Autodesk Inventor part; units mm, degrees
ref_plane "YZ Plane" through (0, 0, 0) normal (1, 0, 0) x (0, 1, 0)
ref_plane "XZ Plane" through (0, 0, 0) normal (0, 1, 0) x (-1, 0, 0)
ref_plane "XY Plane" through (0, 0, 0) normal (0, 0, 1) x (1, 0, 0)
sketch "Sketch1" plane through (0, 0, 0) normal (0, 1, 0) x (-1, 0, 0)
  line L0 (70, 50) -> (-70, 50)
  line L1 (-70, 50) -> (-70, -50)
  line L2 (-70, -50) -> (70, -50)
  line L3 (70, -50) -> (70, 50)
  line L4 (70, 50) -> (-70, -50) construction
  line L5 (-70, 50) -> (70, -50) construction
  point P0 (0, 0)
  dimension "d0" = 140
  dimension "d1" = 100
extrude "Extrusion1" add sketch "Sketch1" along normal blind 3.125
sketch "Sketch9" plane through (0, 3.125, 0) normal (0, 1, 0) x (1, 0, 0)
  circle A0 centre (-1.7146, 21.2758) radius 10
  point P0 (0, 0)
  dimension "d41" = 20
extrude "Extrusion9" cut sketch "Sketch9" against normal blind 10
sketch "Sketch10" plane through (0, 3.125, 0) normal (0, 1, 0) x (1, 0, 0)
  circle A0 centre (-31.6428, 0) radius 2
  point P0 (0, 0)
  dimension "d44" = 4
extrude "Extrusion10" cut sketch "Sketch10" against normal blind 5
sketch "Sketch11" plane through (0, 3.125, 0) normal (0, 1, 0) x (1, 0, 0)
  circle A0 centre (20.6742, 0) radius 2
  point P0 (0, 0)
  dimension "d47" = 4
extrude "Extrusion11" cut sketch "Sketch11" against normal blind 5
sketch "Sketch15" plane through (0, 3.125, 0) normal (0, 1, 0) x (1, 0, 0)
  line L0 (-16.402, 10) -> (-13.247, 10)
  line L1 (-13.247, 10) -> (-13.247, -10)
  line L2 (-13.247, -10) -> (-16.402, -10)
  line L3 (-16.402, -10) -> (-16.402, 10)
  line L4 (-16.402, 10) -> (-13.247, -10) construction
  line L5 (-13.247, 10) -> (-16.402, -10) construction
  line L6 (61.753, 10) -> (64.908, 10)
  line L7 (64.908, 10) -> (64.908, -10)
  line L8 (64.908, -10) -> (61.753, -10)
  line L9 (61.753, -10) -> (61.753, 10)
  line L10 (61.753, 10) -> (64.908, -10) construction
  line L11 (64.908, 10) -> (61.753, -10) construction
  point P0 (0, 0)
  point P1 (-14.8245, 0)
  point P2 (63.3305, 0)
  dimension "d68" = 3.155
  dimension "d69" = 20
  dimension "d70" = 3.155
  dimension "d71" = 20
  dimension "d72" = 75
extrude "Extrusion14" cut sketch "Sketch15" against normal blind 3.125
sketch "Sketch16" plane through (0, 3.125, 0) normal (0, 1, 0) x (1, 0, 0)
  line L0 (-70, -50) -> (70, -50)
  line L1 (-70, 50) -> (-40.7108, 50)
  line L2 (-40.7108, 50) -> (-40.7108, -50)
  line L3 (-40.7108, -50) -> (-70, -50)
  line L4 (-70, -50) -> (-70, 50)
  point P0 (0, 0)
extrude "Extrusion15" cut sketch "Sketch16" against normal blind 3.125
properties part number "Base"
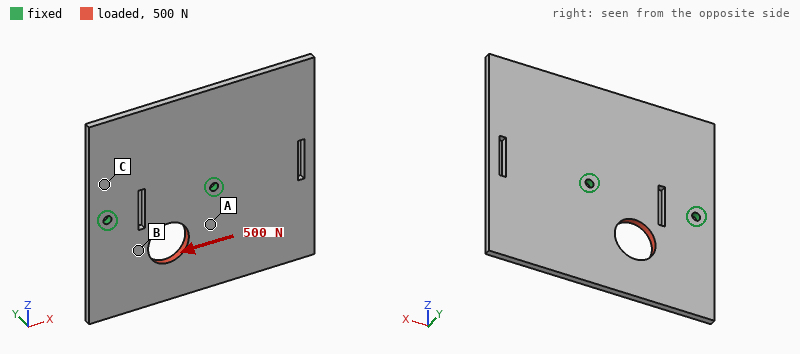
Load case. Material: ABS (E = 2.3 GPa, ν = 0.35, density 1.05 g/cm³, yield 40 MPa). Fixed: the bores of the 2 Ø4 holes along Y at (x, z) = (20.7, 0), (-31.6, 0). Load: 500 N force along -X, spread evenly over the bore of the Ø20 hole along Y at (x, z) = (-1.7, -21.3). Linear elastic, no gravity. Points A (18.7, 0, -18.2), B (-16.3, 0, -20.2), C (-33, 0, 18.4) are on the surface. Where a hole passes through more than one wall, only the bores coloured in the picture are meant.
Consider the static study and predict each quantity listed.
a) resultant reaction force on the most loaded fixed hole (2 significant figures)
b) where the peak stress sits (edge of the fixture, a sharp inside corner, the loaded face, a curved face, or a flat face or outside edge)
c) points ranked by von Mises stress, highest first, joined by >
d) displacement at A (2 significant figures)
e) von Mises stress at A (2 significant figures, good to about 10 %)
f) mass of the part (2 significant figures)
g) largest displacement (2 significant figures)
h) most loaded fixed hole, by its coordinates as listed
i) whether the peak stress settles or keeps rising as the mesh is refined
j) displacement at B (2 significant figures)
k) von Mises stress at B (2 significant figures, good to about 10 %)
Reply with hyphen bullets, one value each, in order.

- 390 N
- edge of the fixture
- B > A > C
- 0.079 mm
- 3.0 MPa
- 35 g
- 0.18 mm
- (20.7, 0)
- keeps rising
- 0.088 mm
- 4.8 MPa
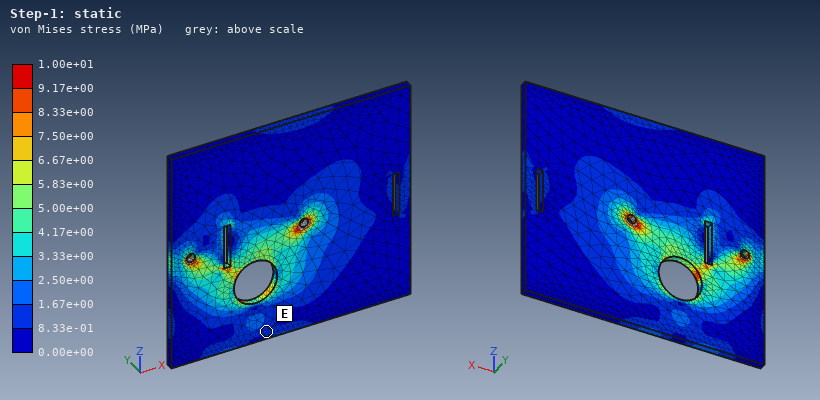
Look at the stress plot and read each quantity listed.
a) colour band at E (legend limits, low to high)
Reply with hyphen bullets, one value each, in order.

- 8.33e-01 to 1.67e+00 MPa
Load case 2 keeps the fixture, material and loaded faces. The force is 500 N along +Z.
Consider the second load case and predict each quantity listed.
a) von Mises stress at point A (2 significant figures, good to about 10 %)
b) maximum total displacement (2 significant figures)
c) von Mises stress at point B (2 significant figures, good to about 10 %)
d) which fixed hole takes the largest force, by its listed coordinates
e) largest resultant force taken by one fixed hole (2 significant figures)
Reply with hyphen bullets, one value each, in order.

- 2.8 MPa
- 74 µm
- 3.4 MPa
- (20.7, 0)
- 290 N
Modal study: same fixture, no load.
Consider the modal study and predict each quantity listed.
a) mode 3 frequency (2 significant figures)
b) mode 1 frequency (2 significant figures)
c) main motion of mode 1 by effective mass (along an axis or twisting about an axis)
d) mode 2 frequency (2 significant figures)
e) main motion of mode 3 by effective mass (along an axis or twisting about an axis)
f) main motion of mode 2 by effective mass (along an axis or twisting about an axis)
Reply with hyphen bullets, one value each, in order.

- 310 Hz
- 190 Hz
- twisting about X
- 230 Hz
- along Y
- along Y
